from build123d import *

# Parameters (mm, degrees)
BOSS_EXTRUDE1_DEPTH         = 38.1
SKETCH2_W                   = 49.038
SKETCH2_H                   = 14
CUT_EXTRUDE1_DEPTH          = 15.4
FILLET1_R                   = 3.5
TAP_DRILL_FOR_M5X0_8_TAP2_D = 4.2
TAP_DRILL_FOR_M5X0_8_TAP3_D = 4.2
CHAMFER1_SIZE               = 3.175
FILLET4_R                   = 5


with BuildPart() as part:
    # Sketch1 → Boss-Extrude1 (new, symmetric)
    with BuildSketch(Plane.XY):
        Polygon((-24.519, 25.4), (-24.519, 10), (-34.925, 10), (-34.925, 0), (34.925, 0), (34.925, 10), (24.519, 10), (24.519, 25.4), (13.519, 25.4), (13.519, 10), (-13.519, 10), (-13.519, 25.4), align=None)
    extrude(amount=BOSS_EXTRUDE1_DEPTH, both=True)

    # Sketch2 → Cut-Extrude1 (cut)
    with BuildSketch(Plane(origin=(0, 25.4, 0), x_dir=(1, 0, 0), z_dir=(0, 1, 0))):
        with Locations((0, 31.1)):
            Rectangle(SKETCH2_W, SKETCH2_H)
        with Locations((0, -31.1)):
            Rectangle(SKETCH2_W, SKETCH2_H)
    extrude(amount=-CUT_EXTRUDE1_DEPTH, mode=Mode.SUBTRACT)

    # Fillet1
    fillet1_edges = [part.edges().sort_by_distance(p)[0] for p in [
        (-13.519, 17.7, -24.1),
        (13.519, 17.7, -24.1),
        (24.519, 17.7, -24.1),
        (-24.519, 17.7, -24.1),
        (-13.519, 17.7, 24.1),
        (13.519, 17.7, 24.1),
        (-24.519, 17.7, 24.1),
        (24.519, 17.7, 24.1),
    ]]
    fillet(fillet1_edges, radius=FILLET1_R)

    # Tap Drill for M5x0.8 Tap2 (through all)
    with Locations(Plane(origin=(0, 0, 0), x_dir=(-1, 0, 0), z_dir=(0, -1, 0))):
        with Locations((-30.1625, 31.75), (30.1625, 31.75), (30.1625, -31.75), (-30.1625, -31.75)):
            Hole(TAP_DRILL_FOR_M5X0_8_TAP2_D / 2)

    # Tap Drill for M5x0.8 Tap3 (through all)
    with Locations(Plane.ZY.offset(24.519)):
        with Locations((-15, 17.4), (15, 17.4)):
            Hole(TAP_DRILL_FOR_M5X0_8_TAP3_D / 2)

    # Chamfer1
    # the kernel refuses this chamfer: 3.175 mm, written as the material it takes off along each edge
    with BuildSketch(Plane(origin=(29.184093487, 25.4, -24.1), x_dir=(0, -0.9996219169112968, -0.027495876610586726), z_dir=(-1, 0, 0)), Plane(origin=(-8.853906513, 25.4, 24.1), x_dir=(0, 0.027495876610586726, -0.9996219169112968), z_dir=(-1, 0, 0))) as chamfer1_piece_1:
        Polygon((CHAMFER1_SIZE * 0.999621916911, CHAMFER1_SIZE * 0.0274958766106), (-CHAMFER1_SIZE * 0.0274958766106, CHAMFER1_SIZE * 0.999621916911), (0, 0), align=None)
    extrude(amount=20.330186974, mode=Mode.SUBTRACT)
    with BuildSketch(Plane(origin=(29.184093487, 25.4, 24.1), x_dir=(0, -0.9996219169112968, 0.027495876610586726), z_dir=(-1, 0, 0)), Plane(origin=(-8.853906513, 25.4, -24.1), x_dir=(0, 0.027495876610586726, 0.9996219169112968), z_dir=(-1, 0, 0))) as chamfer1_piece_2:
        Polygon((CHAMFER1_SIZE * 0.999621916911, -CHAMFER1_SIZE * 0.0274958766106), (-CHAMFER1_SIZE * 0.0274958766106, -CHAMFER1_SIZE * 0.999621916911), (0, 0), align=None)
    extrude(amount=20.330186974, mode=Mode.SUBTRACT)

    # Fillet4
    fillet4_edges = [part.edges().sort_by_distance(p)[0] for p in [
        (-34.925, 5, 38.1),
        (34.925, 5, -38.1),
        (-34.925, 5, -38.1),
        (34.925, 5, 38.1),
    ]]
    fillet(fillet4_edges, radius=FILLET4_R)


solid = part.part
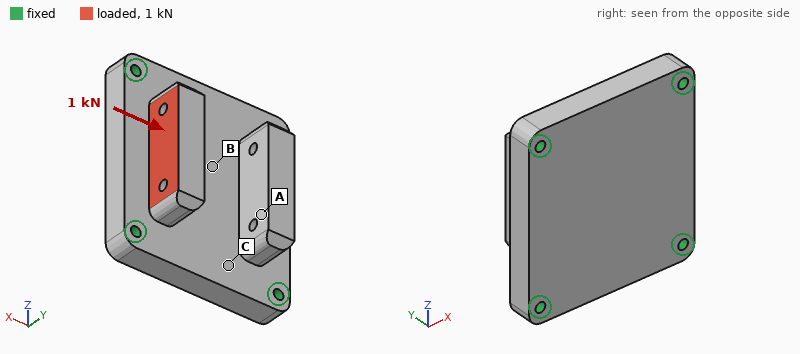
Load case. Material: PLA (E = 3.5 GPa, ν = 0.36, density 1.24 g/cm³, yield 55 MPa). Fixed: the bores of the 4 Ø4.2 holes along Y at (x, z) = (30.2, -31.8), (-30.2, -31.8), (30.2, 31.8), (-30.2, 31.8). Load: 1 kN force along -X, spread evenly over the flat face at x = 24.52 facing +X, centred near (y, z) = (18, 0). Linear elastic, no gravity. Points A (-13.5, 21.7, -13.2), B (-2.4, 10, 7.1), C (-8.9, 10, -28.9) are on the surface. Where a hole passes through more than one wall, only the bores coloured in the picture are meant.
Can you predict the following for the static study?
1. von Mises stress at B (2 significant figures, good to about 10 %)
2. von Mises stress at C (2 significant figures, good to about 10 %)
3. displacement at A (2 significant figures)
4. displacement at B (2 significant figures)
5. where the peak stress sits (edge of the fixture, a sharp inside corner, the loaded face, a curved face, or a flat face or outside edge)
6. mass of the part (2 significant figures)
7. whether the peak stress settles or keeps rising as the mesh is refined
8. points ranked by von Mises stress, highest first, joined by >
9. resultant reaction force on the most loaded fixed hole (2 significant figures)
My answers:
3.8 MPa
2.1 MPa
0.039 mm
0.054 mm
edge of the fixture
84 g
keeps rising
B > C > A
340 N
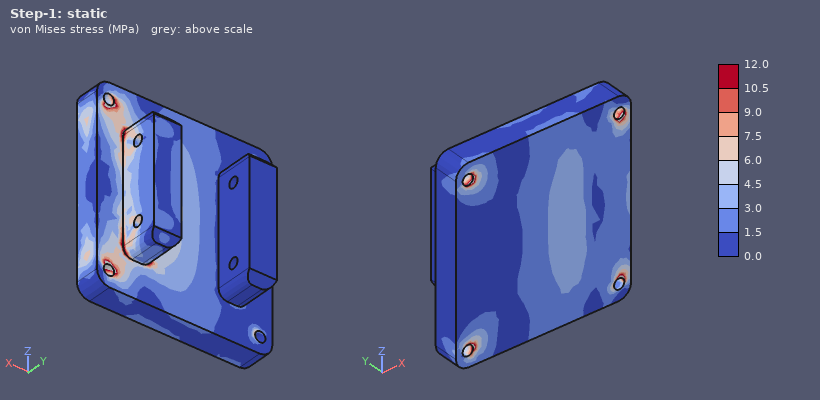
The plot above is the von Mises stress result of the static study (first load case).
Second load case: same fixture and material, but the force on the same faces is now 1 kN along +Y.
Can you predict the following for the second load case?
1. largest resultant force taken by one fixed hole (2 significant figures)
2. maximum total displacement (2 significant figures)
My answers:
480 N
0.14 mm
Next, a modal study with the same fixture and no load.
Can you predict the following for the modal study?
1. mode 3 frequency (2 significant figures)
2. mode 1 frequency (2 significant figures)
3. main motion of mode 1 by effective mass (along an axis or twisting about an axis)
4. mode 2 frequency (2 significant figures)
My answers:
4000 Hz
2400 Hz
along Y
3800 Hz
